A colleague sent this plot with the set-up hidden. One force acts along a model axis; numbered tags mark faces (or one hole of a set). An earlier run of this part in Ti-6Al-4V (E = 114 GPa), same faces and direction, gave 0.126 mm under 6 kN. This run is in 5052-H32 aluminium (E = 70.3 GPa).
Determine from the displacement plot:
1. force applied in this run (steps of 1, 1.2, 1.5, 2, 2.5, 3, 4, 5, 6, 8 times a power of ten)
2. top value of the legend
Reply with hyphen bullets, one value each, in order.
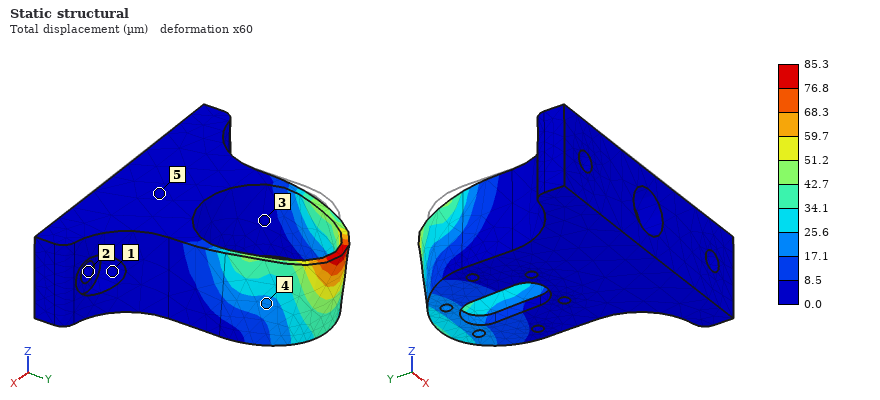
- 2.5 kN
- 85.3 µm
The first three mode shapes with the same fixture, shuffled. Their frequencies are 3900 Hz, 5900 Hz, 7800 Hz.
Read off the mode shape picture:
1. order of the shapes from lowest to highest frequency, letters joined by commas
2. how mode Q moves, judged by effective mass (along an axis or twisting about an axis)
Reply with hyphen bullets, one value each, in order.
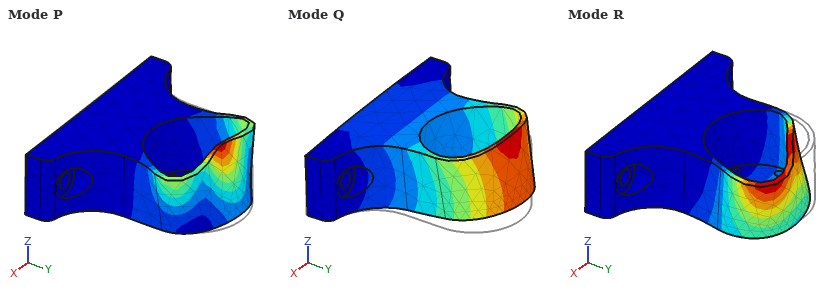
- Q, R, P
- along Z
